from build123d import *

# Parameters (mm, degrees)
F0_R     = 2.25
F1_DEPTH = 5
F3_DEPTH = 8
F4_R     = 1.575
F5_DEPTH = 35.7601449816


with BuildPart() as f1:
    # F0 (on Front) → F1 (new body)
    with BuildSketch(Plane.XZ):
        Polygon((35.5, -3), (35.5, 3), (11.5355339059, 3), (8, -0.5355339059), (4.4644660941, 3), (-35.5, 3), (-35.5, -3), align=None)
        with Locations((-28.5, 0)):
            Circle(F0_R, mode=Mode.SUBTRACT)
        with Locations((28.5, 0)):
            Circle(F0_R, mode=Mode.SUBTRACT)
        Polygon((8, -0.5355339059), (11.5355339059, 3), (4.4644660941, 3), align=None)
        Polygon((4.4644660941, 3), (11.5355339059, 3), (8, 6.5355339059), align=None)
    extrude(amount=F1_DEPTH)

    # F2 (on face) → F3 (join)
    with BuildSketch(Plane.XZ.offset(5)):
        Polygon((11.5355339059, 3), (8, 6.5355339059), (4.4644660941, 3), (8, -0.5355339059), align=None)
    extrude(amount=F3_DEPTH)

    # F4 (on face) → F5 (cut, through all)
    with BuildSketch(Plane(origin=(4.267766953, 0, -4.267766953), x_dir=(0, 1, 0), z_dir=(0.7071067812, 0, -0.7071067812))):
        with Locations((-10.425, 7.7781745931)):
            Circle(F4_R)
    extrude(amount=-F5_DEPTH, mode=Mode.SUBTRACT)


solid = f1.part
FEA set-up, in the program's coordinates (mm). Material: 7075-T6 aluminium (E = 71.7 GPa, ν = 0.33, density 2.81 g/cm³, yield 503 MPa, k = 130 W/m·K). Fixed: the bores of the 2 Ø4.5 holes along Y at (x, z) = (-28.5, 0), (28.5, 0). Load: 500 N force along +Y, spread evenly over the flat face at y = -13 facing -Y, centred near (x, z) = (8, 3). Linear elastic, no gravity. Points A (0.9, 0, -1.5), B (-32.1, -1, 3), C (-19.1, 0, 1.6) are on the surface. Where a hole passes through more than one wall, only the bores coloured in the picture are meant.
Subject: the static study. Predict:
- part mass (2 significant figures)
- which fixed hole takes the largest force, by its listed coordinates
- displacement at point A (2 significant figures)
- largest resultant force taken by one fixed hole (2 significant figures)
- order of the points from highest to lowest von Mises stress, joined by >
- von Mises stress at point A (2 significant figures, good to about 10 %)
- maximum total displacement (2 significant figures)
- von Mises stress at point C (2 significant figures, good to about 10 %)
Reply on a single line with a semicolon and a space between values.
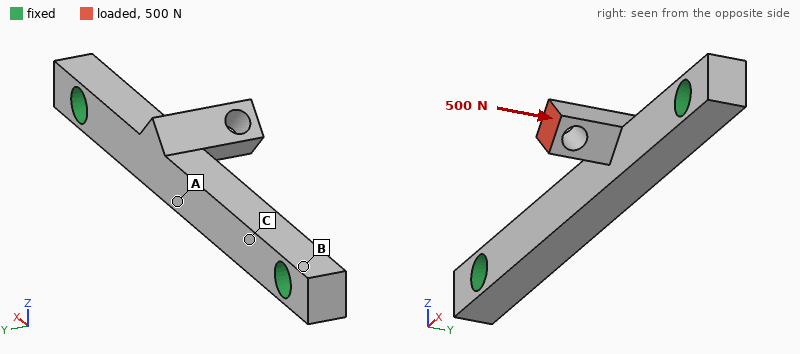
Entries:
6.2 g; (28.5, 0); 0.069 mm; 360 N; A > C > B; 76 MPa; 0.12 mm; 49 MPa
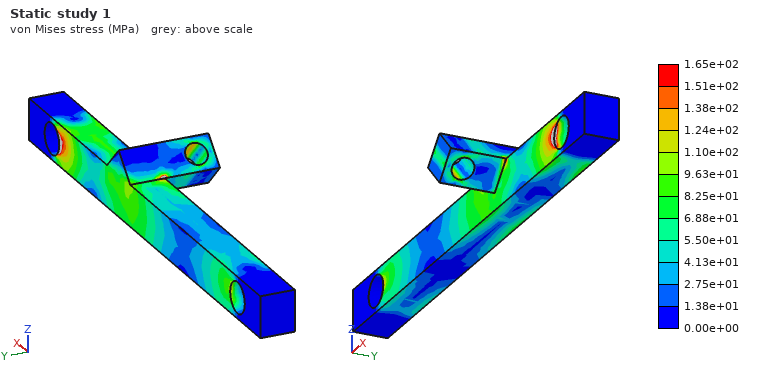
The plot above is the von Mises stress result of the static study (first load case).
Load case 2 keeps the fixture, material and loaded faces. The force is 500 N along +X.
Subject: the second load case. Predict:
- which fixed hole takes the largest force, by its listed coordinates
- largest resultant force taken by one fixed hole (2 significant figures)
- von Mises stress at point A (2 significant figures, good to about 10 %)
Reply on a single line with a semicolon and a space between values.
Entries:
(28.5, 0); 350 N; 80 MPa
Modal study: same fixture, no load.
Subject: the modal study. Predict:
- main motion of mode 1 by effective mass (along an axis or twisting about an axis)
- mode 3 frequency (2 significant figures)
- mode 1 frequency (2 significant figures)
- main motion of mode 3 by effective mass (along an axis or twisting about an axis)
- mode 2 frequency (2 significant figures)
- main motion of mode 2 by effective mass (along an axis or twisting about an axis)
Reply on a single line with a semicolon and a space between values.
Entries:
along Y; 14 kHz; 7700 Hz; twisting about X; 8600 Hz; along Z
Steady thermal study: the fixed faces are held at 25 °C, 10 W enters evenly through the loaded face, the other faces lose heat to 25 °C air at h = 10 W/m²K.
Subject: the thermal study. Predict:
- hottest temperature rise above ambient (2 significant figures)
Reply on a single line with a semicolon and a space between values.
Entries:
74 K
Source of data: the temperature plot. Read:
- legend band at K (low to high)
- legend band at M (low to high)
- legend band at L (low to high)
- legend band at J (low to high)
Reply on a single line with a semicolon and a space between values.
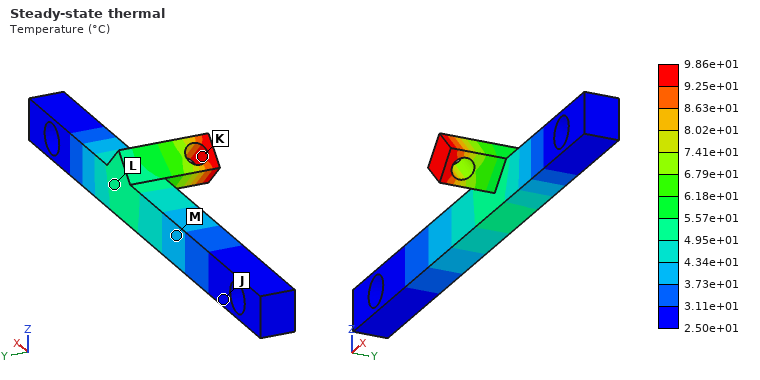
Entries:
9.25e+01 to 9.86e+01 °C; 3.73e+01 to 4.34e+01 °C; 4.95e+01 to 5.57e+01 °C; 2.50e+01 to 3.11e+01 °C
